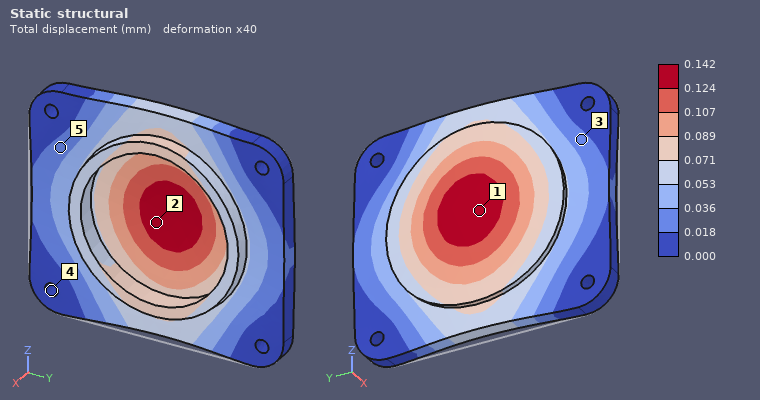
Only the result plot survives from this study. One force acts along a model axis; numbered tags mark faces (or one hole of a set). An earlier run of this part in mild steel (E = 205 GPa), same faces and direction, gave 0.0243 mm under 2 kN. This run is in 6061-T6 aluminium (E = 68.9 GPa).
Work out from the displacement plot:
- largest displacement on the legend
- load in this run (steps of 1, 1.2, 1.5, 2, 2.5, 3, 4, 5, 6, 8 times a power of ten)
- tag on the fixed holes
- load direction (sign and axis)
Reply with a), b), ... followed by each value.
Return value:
a) 0.142 mm
b) 4 kN
c) 4
d) -X
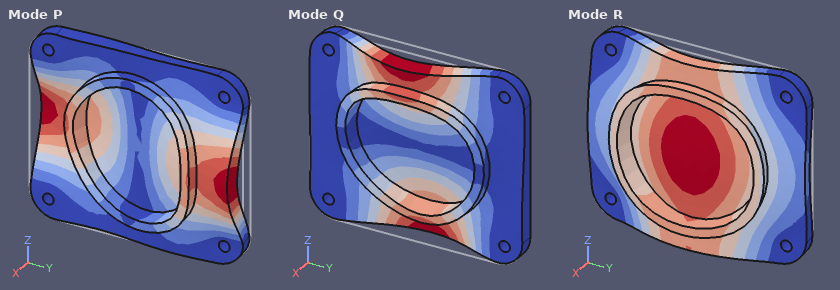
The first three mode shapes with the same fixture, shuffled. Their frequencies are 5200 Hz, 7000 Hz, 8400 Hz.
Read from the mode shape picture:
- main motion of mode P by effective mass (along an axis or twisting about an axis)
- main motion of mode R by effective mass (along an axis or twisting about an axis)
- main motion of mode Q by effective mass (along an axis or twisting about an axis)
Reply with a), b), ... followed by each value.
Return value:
a) twisting about Z
b) along X
c) twisting about Y
